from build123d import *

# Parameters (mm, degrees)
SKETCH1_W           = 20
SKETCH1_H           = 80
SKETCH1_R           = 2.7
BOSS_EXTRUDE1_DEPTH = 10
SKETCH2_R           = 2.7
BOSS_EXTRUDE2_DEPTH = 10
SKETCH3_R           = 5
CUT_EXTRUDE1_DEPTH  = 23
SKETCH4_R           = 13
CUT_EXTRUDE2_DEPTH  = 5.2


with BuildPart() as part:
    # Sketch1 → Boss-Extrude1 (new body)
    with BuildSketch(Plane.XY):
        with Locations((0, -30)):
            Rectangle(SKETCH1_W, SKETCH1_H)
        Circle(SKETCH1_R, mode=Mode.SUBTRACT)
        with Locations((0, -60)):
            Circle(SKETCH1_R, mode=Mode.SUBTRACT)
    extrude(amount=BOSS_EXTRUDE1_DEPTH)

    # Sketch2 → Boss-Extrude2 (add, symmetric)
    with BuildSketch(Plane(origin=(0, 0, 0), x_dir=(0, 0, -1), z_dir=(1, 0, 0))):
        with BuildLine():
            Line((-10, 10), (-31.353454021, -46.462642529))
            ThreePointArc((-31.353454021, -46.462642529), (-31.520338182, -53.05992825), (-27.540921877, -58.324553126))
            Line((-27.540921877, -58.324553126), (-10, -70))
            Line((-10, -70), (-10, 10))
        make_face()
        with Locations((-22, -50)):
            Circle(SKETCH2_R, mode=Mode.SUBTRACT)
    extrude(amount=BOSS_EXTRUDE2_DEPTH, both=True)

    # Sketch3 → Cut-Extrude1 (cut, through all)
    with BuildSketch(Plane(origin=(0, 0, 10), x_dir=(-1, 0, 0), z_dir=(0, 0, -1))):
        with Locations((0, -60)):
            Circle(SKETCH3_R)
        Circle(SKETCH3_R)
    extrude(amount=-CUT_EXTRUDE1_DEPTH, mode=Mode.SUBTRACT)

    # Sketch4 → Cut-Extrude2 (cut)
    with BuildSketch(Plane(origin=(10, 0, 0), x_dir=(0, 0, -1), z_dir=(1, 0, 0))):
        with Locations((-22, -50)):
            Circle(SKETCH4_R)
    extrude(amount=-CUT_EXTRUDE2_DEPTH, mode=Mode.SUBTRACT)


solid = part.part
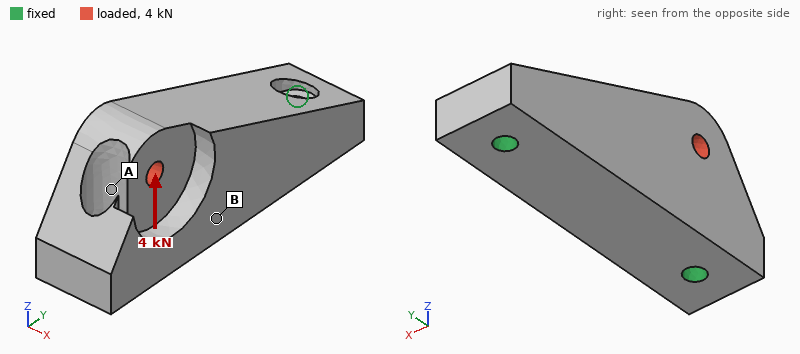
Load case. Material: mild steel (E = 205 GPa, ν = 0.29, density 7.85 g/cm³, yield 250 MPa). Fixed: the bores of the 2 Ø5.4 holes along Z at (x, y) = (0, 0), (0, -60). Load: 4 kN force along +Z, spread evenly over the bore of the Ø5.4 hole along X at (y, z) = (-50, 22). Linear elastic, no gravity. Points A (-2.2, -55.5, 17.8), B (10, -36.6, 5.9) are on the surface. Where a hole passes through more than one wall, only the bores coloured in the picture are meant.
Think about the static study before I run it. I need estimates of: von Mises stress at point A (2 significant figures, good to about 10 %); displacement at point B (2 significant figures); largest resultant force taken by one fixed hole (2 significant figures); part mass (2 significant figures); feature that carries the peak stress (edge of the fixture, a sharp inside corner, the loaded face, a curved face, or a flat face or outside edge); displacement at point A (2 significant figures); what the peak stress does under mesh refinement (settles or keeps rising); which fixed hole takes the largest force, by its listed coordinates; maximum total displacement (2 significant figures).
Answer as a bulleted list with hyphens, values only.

- 26 MPa
- 1.8 µm
- 3.5 kN
- 240 g
- edge of the fixture
- 2.9 µm
- keeps rising
- (0, -60)
- 4.0 µm
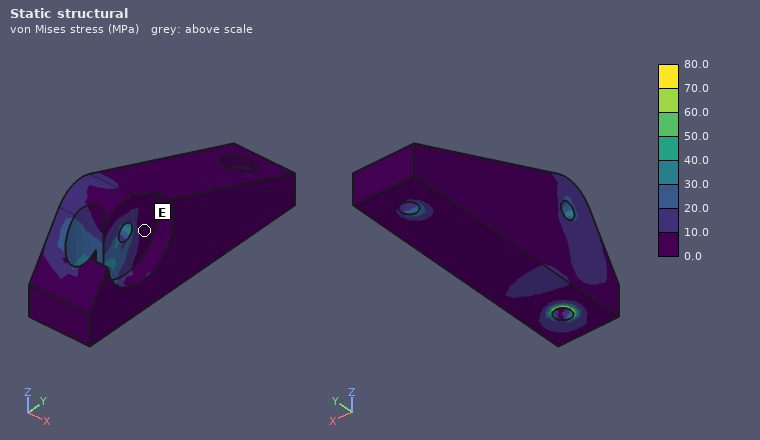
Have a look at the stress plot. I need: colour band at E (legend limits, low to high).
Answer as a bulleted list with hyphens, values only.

- 0.0 to 10.0 MPa
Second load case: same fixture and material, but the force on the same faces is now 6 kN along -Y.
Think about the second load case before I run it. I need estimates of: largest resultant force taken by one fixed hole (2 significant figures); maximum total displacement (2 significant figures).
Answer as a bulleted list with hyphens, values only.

- 3.4 kN
- 5.7 µm
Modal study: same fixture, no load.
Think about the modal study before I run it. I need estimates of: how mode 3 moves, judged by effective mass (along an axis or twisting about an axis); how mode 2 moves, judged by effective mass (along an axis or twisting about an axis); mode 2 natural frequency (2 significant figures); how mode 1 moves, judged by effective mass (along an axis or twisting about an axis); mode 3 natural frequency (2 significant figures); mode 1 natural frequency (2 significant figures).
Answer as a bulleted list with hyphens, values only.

- along X
- along Z
- 14 kHz
- along X
- 16 kHz
- 8500 Hz
